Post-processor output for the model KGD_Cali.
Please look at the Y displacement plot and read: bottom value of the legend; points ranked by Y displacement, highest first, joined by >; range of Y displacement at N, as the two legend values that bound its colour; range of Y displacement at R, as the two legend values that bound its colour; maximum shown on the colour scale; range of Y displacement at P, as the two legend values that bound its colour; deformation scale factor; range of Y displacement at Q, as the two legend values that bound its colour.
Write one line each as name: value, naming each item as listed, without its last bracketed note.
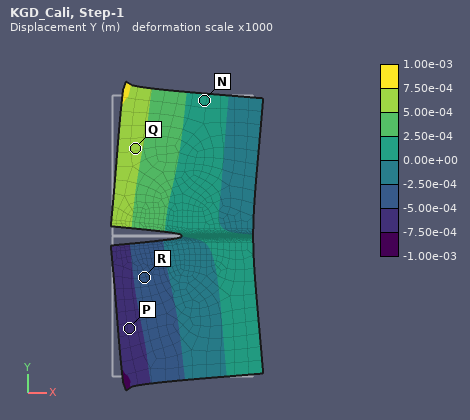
bottom value of the legend: -1.00e-03 m
points ranked by Y displacement, highest first, joined by >: Q > N > R > P
range of Y displacement at N, as the two legend values that bound its colour: 0.00e+00 to 2.50e-04 m
range of Y displacement at R, as the two legend values that bound its colour: -5.00e-04 to -2.50e-04 m
maximum shown on the colour scale: 1.00e-03 m
range of Y displacement at P, as the two legend values that bound its colour: -7.50e-04 to -5.00e-04 m
deformation scale factor: 1000
range of Y displacement at Q, as the two legend values that bound its colour: 5.00e-04 to 7.50e-04 m
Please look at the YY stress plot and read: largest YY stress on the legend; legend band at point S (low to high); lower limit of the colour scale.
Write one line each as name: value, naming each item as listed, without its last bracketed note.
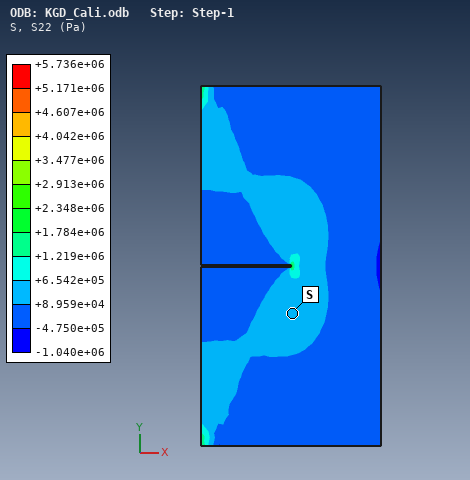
largest YY stress on the legend: +5.736e+06 Pa
legend band at point S: +8.959e+04 to +6.542e+05 Pa
lower limit of the colour scale: -1.040e+06 Pa
